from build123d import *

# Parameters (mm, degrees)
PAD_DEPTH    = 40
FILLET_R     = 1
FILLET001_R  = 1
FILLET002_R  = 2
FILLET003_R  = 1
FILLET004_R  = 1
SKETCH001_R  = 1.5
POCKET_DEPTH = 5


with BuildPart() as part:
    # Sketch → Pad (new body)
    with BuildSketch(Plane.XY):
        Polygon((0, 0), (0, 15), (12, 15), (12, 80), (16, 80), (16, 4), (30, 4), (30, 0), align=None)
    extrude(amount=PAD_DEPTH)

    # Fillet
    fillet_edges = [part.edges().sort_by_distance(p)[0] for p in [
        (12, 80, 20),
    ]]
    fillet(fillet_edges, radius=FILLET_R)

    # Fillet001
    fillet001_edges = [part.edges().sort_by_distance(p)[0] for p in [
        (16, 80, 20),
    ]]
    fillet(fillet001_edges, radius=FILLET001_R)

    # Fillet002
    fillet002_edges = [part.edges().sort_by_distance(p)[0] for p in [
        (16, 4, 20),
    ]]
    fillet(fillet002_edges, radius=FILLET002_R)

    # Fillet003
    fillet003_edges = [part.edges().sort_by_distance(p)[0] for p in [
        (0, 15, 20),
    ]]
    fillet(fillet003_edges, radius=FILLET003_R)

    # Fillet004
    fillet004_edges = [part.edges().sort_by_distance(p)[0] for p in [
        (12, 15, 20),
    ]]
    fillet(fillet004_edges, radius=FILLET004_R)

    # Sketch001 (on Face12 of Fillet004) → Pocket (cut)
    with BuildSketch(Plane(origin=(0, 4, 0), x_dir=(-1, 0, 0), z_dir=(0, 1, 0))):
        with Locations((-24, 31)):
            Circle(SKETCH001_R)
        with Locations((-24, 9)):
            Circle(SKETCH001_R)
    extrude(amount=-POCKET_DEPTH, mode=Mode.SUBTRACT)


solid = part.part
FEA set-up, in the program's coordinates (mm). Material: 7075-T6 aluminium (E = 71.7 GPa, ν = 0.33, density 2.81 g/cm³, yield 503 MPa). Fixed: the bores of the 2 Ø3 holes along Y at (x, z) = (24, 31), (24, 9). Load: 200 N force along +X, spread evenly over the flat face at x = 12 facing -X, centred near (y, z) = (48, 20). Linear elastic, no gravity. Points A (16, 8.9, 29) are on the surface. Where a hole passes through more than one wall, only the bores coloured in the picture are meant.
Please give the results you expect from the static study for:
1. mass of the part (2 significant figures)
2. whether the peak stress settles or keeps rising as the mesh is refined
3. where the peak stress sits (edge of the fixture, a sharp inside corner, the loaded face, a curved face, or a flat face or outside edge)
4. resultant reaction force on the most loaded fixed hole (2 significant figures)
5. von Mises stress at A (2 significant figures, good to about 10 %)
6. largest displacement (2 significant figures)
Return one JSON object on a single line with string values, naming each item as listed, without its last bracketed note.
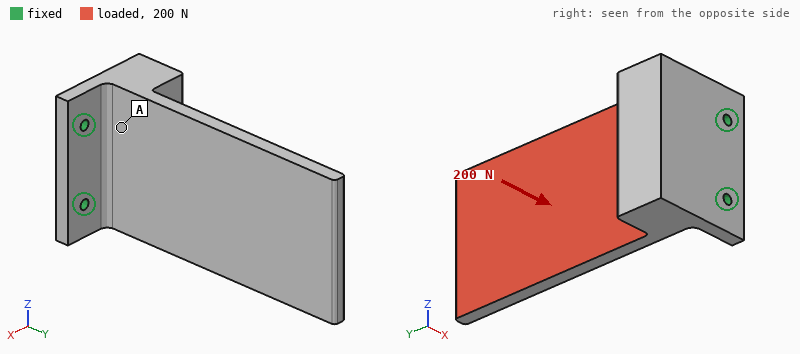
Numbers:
{"mass of the part": "62 g", "whether the peak stress settles or keeps rising as the mesh is refined": "keeps rising", "where the peak stress sits": "edge of the fixture", "resultant reaction force on the most loaded fixed hole": "110 N", "von Mises stress at A": "12 MPa", "largest displacement": "0.94 mm"}
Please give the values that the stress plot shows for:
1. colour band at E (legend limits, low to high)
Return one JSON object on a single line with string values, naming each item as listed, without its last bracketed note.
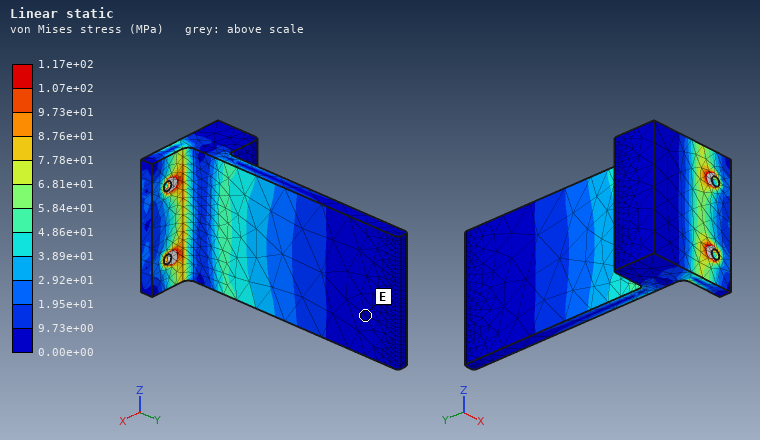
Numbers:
{"colour band at E": "0.00e+00 to 9.73e+00 MPa"}
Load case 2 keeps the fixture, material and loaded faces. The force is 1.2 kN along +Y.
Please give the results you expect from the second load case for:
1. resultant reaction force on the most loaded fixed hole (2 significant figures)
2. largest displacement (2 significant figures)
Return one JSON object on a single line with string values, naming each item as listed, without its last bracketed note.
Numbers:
{"resultant reaction force on the most loaded fixed hole": "600 N", "largest displacement": "0.71 mm"}
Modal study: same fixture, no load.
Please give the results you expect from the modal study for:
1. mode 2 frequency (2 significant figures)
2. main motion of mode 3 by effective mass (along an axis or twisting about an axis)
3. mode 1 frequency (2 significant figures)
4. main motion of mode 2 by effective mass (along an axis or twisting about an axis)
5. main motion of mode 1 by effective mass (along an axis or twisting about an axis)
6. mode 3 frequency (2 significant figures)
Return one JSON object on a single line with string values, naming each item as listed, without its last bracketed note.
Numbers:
{"mode 2 frequency": "2000 Hz", "main motion of mode 3 by effective mass": "along Y", "mode 1 frequency": "530 Hz", "main motion of mode 2 by effective mass": "along Z", "main motion of mode 1 by effective mass": "along X", "mode 3 frequency": "2400 Hz"}
